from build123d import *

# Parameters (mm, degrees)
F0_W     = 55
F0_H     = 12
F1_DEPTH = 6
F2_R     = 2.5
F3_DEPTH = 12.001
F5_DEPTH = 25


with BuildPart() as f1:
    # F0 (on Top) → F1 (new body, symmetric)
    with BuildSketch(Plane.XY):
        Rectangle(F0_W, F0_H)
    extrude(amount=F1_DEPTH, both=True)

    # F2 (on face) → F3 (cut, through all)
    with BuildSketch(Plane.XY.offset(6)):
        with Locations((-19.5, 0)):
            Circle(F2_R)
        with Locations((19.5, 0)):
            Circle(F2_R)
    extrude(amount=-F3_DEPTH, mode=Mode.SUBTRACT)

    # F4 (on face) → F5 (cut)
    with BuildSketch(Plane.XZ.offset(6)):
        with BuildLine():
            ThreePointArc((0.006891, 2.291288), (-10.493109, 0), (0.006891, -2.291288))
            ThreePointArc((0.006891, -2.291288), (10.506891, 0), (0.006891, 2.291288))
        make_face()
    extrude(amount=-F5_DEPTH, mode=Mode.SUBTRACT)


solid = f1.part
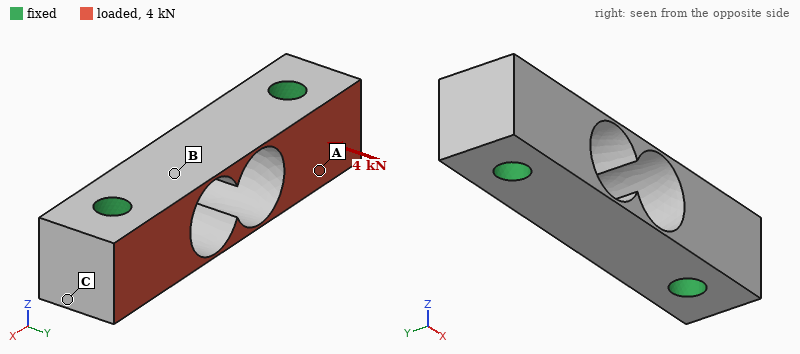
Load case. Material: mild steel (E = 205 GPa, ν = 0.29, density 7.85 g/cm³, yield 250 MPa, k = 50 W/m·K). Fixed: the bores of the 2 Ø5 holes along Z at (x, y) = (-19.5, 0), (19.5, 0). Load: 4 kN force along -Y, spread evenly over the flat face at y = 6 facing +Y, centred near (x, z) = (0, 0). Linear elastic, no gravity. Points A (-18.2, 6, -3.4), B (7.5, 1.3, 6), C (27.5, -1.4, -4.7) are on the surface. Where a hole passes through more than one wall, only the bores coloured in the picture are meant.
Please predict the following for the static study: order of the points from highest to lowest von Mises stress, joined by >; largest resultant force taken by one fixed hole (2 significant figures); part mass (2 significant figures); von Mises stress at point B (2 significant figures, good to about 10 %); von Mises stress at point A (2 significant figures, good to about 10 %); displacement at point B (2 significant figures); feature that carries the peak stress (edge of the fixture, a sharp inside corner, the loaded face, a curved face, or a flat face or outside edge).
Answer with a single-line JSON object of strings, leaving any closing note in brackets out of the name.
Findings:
{"order of the points from highest to lowest von Mises stress, joined by >": "A > B > C", "largest resultant force taken by one fixed hole": "2.0 kN", "part mass": "41 g", "von Mises stress at point B": "13 MPa", "von Mises stress at point A": "23 MPa", "displacement at point B": "1.8 µm", "feature that carries the peak stress": "the loaded face"}
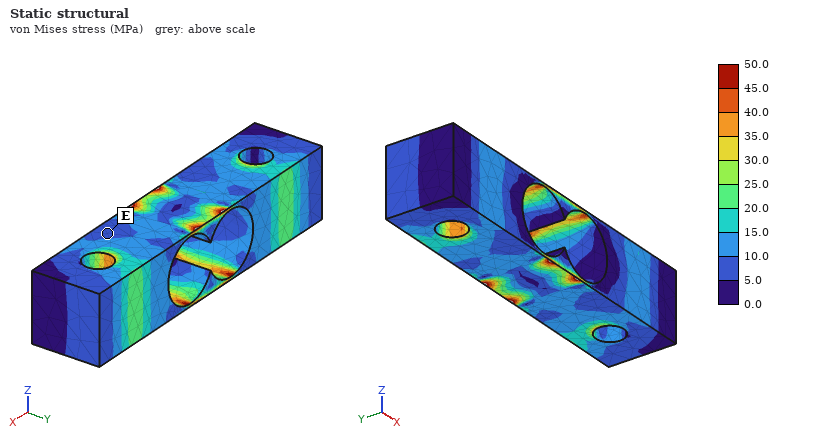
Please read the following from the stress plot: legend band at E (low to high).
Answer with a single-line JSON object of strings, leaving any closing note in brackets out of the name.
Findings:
{"legend band at E": "5.0 to 10.0 MPa"}
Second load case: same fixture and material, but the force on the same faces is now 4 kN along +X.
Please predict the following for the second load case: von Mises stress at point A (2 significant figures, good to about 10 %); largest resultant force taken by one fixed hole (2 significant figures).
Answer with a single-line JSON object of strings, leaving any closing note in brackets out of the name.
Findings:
{"von Mises stress at point A": "15 MPa", "largest resultant force taken by one fixed hole": "2.0 kN"}
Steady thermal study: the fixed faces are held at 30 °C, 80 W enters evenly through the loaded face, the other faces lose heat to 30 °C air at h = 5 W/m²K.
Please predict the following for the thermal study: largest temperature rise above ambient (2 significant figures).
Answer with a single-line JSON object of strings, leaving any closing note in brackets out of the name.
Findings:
{"largest temperature rise above ambient": "53 K"}
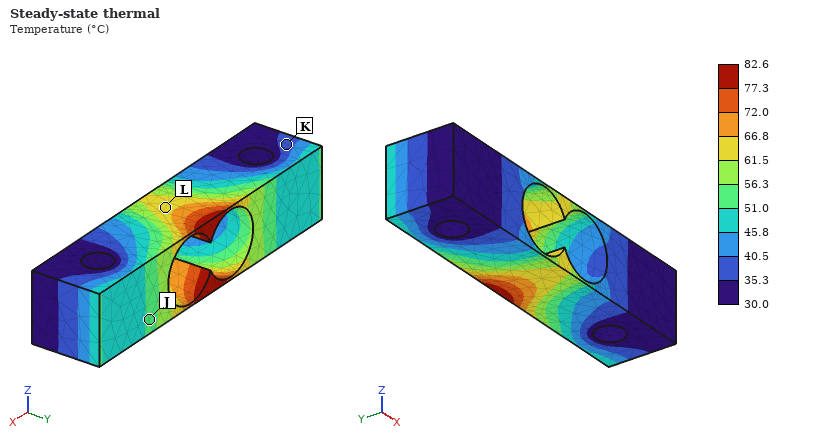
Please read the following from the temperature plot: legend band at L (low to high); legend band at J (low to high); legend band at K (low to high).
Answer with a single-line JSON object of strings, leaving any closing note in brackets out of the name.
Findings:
{"legend band at L": "61.5 to 66.8 °C", "legend band at J": "51.0 to 56.3 °C", "legend band at K": "35.3 to 40.5 °C"}
